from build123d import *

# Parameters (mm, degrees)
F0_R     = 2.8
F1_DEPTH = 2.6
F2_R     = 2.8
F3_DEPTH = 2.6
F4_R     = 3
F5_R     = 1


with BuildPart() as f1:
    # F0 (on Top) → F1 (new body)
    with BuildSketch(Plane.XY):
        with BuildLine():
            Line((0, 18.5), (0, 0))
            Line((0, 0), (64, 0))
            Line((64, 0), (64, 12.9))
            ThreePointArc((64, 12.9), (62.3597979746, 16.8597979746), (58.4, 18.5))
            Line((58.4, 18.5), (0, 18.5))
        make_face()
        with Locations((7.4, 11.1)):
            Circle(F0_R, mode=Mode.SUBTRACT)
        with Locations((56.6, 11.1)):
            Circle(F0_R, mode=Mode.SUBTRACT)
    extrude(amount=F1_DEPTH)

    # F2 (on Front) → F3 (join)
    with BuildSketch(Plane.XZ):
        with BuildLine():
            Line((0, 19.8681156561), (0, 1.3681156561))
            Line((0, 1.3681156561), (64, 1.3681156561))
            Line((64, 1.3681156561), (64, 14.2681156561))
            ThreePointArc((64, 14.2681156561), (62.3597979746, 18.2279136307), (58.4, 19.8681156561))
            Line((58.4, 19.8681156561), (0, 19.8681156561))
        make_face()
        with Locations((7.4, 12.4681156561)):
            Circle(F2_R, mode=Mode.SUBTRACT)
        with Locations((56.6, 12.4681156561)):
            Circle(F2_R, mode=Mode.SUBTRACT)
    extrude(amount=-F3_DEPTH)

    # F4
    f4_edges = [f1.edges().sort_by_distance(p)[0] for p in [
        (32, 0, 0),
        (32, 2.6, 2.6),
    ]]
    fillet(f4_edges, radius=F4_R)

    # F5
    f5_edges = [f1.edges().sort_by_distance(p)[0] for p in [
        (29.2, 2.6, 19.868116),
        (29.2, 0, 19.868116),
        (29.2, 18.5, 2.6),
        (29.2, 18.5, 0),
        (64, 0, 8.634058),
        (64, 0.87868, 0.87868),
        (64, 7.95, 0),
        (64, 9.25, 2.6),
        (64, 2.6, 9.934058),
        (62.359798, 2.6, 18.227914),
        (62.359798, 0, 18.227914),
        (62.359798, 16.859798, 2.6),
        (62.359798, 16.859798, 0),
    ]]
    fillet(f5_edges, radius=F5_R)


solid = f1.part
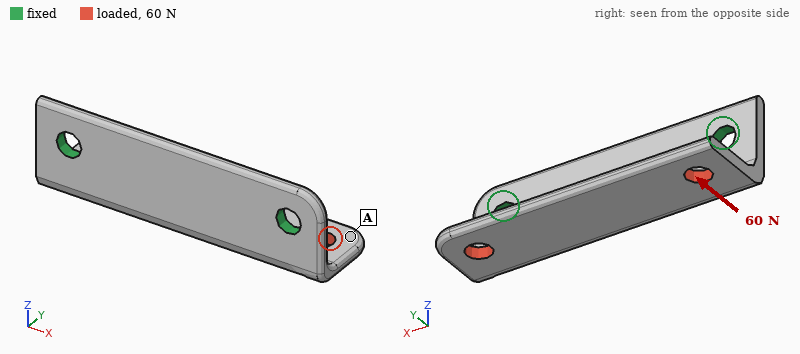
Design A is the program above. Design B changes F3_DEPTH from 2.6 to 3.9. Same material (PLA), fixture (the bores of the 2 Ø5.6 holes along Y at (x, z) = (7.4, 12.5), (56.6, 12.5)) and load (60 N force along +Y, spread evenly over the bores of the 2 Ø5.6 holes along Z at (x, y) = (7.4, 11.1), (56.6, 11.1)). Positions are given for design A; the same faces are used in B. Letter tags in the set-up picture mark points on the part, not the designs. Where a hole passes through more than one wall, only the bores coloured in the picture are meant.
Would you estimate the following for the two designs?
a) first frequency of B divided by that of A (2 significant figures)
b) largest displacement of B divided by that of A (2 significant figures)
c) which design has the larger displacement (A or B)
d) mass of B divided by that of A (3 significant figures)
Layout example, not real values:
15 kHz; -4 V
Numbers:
1.6; 0.34; A; 1.24
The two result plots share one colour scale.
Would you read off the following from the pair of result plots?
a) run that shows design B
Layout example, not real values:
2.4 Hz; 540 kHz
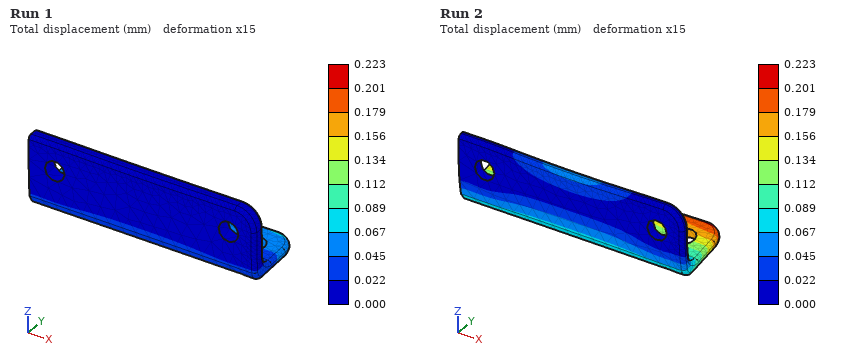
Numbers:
Run 1
